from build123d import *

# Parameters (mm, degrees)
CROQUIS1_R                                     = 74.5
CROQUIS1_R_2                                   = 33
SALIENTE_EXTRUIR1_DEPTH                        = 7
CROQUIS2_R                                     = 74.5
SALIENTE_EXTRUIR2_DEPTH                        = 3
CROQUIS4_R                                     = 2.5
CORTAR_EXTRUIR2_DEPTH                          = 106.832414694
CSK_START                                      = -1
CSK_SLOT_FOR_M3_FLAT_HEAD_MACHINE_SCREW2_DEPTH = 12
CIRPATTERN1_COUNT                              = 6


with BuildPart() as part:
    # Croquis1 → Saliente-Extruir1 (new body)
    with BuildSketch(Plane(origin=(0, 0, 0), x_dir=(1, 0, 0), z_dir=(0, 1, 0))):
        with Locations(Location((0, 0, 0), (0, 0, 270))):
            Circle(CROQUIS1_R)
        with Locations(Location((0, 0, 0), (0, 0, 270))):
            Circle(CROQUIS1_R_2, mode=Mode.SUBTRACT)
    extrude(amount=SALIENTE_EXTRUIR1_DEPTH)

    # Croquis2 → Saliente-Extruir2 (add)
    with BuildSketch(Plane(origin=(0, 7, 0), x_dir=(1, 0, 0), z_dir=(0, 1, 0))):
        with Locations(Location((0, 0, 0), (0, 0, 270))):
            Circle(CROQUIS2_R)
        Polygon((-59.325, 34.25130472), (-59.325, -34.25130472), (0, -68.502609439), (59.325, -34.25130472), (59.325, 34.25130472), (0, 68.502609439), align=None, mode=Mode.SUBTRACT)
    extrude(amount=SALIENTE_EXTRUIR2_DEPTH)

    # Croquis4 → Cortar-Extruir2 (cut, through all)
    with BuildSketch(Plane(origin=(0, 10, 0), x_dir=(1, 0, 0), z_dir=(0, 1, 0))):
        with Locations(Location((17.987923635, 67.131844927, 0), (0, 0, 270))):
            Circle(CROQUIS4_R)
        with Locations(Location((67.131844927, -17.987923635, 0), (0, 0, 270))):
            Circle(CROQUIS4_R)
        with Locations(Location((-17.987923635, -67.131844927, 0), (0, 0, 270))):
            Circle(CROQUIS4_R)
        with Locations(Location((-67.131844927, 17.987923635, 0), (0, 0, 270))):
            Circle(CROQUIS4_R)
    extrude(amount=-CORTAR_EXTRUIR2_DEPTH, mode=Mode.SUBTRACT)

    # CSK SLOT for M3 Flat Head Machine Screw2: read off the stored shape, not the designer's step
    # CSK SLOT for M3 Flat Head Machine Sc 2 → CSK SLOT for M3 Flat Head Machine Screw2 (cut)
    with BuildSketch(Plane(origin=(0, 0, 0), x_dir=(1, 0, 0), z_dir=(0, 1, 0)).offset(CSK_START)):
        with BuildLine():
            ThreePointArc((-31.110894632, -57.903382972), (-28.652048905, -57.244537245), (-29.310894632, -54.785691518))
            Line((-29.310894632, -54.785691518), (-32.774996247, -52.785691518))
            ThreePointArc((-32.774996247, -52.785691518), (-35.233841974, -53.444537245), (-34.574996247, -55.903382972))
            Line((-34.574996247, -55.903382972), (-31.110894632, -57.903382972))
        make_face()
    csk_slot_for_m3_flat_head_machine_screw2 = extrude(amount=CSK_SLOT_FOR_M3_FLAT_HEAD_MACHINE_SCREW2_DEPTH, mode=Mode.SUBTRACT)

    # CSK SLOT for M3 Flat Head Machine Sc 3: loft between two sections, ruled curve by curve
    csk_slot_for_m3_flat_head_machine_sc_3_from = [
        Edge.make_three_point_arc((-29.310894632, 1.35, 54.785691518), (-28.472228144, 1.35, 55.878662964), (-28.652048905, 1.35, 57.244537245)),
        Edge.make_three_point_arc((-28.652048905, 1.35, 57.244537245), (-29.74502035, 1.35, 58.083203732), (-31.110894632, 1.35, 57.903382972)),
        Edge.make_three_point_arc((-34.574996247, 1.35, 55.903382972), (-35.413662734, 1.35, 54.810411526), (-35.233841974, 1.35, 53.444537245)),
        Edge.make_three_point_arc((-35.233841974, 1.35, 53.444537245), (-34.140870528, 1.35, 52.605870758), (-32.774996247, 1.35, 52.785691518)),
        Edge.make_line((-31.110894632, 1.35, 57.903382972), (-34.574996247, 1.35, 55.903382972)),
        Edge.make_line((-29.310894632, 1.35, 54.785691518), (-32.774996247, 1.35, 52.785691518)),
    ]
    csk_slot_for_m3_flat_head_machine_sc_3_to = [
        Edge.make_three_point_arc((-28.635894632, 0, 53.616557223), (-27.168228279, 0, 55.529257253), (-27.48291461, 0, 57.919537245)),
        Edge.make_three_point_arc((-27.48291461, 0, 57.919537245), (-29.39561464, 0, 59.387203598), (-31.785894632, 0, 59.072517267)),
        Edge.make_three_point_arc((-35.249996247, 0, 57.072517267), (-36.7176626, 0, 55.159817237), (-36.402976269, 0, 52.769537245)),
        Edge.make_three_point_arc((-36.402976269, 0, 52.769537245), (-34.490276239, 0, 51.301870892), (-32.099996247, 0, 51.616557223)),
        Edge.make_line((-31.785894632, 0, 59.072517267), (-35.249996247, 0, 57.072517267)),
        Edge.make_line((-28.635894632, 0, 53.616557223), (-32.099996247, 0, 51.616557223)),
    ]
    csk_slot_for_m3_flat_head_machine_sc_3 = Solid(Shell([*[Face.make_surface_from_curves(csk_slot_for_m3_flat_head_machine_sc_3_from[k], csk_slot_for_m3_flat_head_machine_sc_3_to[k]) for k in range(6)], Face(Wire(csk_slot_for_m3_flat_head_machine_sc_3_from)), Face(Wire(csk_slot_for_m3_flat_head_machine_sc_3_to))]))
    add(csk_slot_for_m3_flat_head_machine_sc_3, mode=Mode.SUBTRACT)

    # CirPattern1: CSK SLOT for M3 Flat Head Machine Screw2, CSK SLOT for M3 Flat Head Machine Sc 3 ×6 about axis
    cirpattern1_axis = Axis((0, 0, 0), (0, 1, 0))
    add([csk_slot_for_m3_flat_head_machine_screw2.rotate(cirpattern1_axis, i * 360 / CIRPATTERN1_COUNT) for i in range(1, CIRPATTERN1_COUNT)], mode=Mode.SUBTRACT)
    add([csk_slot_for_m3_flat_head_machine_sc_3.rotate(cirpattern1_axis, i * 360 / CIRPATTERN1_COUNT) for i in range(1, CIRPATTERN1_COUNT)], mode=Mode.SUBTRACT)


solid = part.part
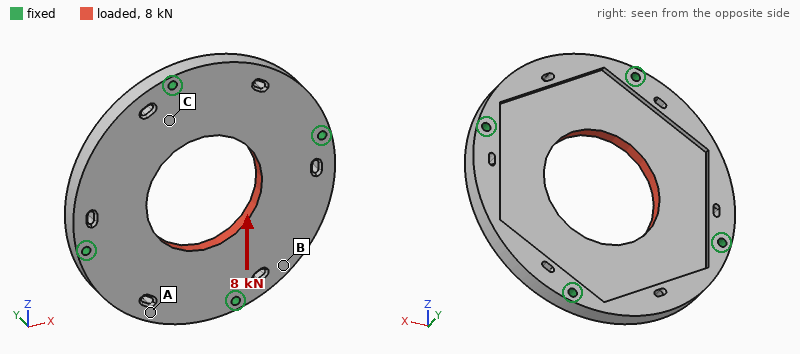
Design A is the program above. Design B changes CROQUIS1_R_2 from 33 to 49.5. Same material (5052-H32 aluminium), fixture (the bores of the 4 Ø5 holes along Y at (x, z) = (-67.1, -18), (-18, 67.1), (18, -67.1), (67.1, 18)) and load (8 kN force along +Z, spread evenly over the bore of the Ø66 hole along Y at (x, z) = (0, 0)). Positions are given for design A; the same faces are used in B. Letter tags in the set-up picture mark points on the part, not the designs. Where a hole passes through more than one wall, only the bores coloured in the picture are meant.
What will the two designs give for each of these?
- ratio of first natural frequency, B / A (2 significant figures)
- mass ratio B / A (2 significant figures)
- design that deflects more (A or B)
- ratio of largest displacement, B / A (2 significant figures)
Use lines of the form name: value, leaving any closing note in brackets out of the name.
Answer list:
ratio of first natural frequency, B / A: 1.0
mass ratio B / A: 0.73
design that deflects more: B
ratio of largest displacement, B / A: 1.3
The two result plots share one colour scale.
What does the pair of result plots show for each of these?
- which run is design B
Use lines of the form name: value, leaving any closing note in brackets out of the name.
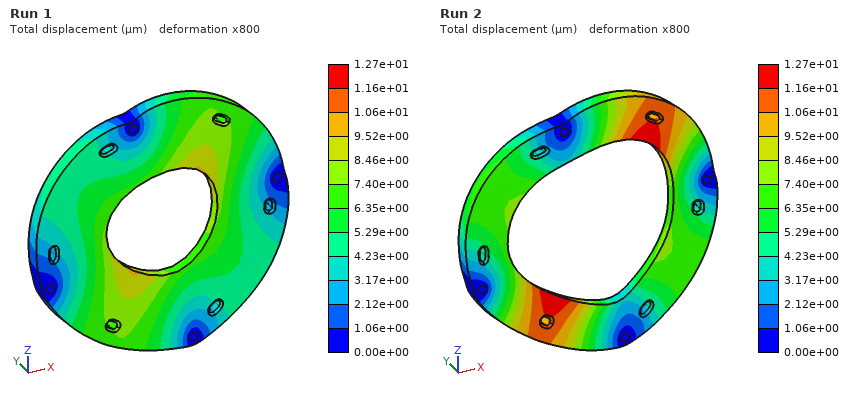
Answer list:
which run is design B: Run 2
